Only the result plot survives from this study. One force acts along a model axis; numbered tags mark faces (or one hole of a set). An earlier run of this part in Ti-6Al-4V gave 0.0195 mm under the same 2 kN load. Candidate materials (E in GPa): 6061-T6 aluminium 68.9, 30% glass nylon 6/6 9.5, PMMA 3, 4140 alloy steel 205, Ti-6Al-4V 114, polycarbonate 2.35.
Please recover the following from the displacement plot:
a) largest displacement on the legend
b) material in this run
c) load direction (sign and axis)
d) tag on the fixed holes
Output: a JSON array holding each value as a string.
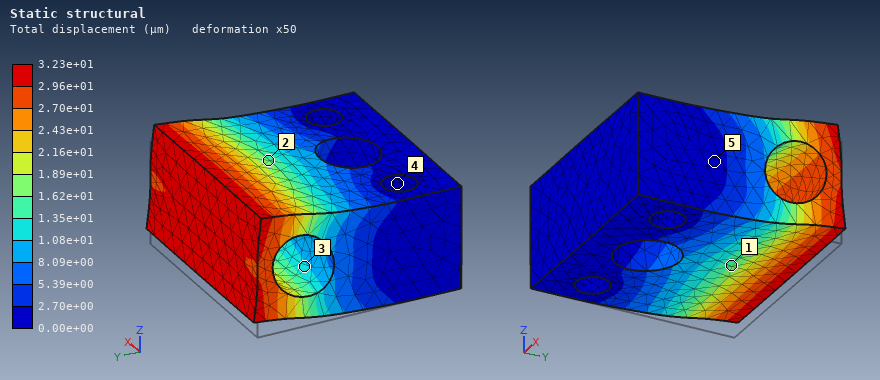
["3.23e+01 µm", "6061-T6 aluminium", "+Z", "4"]
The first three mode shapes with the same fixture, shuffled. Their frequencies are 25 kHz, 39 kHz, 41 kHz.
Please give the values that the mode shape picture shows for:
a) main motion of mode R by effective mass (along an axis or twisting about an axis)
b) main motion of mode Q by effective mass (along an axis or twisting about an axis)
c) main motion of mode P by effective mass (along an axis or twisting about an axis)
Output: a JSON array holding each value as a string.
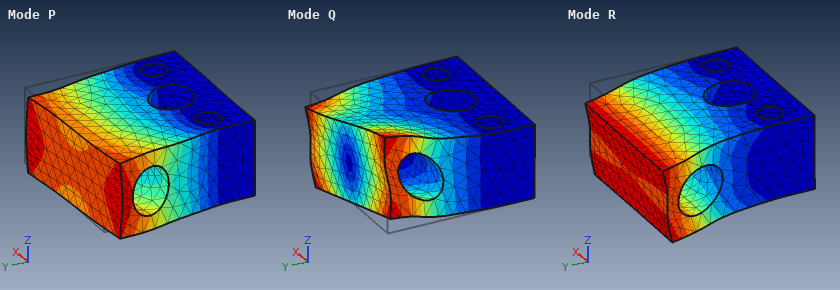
["along Z", "twisting about Y", "along X"]
